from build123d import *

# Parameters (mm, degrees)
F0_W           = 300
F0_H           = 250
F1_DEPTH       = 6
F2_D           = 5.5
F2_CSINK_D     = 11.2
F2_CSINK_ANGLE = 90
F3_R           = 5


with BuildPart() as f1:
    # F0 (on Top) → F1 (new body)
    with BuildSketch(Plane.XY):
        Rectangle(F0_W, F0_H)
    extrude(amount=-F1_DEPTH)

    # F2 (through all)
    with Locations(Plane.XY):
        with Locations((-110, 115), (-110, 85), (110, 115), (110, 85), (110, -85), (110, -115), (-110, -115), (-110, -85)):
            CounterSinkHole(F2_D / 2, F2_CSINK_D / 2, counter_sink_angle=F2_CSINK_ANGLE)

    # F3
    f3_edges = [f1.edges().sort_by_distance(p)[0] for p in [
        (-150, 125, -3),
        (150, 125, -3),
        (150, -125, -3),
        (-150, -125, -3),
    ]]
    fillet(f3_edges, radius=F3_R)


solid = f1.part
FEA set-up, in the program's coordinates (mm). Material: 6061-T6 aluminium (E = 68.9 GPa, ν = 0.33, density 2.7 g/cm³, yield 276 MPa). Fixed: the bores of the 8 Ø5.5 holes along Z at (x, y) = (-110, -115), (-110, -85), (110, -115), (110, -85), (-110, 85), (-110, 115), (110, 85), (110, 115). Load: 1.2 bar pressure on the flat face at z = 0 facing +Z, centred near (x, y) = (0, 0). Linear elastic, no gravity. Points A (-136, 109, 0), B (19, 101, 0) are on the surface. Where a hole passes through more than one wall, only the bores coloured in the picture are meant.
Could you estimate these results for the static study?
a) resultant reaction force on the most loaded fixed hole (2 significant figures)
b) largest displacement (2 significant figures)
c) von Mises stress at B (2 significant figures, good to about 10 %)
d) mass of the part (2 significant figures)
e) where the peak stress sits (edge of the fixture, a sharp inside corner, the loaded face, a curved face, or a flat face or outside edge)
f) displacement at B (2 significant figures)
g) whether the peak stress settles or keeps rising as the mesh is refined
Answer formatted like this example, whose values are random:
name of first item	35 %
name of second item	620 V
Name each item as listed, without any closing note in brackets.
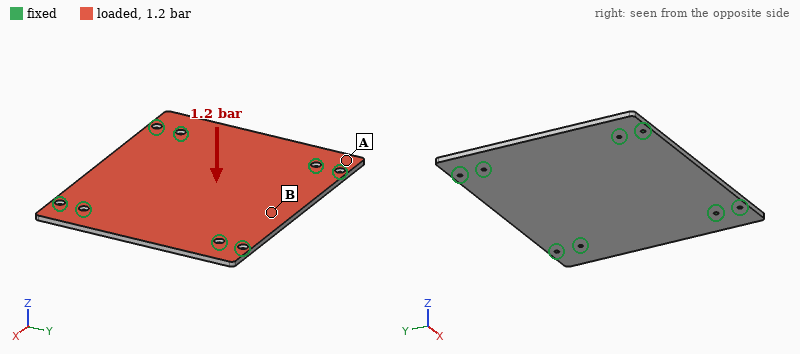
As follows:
resultant reaction force on the most loaded fixed hole	3.2 kN
largest displacement	1.2 mm
von Mises stress at B	52 MPa
mass of the part	1.2 kg
where the peak stress sits	edge of the fixture
displacement at B	0.86 mm
whether the peak stress settles or keeps rising as the mesh is refined	keeps rising
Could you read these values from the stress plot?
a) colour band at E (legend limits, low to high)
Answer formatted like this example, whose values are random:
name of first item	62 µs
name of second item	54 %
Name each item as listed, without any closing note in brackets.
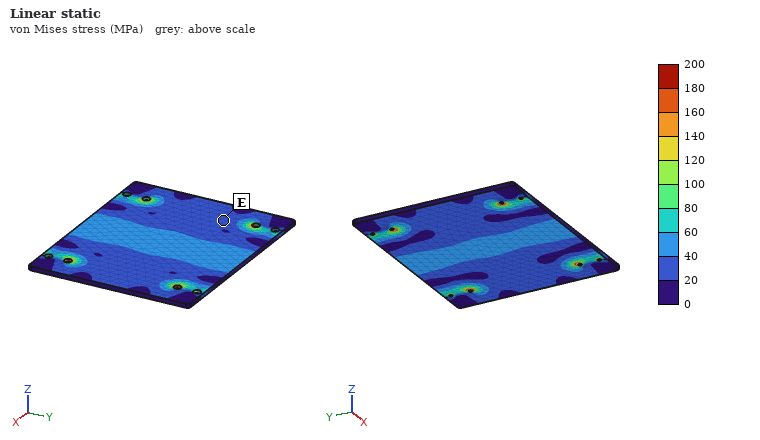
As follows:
colour band at E	20 to 40 MPa
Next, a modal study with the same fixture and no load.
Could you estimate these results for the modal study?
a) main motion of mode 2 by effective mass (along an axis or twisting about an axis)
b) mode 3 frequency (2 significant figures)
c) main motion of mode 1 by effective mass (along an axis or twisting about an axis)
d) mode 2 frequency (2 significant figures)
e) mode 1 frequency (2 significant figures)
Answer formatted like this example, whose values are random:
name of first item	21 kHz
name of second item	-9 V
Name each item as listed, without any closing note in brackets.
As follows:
main motion of mode 2 by effective mass	twisting about X
mode 3 frequency	860 Hz
main motion of mode 1 by effective mass	along Z
mode 2 frequency	680 Hz
mode 1 frequency	460 Hz
